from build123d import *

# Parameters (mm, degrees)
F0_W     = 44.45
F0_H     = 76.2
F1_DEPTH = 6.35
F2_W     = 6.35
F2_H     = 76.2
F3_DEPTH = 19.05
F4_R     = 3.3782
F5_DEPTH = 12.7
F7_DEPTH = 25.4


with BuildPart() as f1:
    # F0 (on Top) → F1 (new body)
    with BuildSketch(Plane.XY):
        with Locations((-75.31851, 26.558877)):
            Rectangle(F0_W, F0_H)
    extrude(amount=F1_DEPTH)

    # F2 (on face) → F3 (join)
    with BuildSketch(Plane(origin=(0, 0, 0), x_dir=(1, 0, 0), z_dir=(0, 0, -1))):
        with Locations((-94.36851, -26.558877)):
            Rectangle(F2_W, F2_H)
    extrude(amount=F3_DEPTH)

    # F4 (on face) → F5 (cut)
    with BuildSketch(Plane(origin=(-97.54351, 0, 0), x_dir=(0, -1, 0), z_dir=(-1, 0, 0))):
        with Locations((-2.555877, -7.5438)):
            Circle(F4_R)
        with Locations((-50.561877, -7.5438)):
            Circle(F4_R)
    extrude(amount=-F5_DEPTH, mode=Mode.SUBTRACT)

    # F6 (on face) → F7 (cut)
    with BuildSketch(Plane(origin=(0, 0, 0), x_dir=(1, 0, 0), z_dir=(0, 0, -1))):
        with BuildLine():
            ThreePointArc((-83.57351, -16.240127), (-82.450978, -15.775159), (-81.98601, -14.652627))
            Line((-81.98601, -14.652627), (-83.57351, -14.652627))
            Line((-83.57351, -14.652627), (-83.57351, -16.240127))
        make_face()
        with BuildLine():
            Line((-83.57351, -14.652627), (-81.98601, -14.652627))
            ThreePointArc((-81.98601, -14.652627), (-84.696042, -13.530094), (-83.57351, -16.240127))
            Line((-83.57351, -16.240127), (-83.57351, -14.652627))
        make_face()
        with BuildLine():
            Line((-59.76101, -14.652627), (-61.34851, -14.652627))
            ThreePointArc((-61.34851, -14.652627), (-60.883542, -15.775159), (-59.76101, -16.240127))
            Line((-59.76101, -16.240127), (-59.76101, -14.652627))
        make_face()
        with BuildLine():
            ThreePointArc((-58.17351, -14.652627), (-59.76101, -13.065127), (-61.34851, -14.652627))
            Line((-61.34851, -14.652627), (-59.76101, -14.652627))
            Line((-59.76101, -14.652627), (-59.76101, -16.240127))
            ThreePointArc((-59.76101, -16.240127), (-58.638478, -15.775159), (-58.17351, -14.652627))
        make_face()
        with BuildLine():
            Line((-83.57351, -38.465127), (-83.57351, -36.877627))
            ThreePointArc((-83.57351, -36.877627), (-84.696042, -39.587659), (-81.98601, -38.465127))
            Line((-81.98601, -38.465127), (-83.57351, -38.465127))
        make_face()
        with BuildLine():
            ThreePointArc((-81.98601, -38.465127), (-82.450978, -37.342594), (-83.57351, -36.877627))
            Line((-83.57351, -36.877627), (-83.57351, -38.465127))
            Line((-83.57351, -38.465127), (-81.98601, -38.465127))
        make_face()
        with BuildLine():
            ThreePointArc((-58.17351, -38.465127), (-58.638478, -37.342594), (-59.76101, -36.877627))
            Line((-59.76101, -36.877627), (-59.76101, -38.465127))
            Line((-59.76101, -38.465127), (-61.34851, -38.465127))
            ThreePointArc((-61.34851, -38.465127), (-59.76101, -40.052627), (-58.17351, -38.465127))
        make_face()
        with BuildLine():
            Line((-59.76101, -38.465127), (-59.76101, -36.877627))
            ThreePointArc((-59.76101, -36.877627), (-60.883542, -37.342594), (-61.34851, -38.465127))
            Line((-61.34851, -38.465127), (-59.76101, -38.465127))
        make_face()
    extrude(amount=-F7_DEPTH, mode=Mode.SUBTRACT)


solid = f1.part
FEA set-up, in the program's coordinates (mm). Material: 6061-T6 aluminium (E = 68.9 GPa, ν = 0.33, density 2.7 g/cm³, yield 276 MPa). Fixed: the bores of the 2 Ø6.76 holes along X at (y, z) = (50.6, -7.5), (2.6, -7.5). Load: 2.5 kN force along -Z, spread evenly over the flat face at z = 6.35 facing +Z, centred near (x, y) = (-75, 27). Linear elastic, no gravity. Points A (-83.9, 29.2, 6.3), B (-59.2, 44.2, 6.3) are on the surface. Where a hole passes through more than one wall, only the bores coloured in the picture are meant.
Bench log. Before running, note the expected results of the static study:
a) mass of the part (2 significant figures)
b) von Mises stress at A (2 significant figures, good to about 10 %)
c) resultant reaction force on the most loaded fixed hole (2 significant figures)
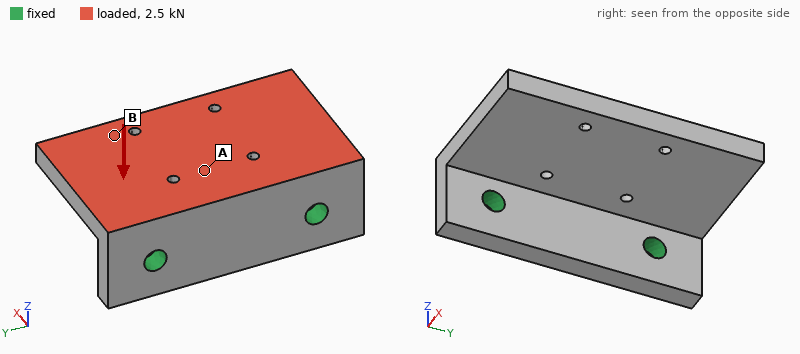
81 g
47 MPa
1.3 kN
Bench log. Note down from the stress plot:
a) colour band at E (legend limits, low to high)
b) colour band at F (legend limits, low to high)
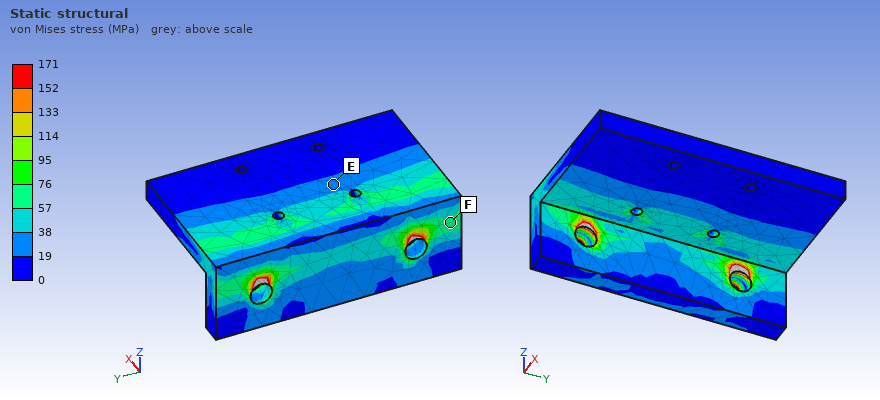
19 to 38 MPa
57 to 76 MPa
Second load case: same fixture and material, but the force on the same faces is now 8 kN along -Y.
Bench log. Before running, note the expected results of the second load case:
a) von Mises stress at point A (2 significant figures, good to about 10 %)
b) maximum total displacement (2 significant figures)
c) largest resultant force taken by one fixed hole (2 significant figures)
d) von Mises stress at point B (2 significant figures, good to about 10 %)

27 MPa
72 µm
5.3 kN
14 MPa
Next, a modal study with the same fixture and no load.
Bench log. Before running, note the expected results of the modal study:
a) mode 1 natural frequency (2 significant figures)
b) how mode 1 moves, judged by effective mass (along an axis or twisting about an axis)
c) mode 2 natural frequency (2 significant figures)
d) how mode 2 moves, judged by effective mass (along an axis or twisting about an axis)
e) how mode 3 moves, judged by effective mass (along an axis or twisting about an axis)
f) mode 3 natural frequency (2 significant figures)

2200 Hz
along Z
4000 Hz
twisting about X
along Y
7900 Hz
